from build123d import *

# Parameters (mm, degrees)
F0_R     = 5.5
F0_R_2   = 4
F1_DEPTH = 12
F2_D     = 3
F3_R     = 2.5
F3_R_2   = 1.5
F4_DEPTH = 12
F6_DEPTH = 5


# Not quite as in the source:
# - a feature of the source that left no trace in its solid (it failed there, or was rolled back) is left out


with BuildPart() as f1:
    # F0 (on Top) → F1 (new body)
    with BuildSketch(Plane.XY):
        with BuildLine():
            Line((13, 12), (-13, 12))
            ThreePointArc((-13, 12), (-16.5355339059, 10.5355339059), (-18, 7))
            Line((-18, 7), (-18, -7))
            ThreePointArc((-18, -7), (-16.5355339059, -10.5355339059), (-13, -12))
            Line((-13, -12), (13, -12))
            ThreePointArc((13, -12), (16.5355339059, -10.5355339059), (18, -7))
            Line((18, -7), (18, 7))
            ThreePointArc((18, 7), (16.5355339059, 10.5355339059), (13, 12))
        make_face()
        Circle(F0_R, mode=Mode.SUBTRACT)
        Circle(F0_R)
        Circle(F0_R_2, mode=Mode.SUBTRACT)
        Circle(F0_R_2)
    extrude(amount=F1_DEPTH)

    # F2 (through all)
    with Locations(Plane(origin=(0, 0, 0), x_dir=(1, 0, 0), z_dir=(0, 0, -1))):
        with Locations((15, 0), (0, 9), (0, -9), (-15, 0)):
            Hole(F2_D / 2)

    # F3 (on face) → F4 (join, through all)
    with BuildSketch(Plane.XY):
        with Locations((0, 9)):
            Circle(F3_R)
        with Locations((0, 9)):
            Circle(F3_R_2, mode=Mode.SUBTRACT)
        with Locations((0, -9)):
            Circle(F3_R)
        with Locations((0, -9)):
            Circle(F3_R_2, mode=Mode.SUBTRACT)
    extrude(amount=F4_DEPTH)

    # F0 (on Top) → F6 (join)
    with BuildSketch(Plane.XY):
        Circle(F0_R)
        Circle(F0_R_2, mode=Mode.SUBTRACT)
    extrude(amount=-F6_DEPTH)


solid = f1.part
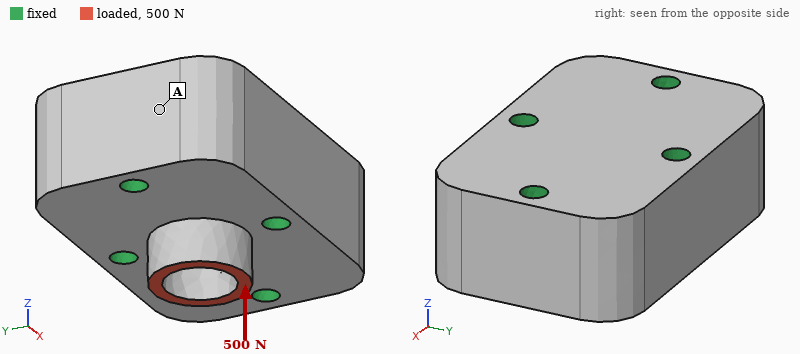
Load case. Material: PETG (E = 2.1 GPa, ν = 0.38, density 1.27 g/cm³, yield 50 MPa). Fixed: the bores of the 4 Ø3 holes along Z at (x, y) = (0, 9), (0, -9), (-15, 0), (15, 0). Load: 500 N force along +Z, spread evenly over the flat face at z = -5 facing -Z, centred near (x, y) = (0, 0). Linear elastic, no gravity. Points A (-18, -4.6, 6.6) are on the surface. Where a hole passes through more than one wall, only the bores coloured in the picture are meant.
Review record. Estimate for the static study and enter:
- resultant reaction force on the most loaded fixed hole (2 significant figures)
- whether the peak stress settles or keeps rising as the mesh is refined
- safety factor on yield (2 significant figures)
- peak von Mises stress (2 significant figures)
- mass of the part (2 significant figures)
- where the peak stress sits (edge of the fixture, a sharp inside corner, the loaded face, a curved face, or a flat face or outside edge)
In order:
180 N
settles
3.9
13 MPa
13 g
a curved face
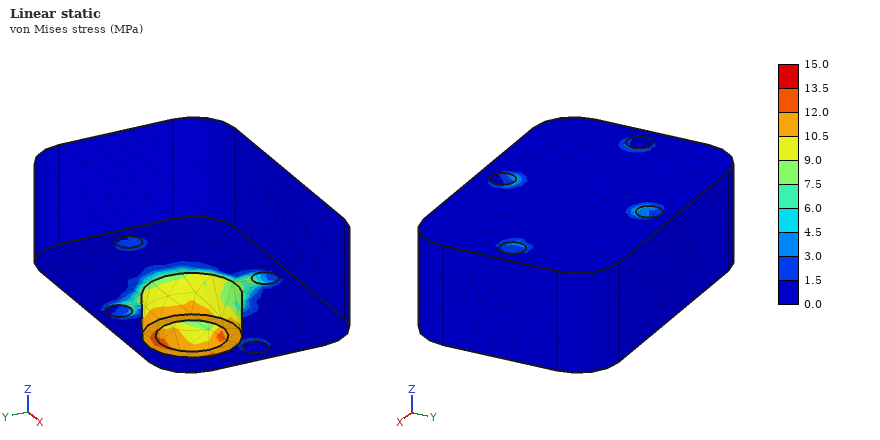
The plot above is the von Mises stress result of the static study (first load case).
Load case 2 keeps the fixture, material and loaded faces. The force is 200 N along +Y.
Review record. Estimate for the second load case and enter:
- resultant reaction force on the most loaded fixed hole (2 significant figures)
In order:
120 N
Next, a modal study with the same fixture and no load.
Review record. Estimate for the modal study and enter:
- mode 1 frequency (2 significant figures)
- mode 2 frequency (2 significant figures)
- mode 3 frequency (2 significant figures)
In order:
14 kHz
14 kHz
14 kHz
